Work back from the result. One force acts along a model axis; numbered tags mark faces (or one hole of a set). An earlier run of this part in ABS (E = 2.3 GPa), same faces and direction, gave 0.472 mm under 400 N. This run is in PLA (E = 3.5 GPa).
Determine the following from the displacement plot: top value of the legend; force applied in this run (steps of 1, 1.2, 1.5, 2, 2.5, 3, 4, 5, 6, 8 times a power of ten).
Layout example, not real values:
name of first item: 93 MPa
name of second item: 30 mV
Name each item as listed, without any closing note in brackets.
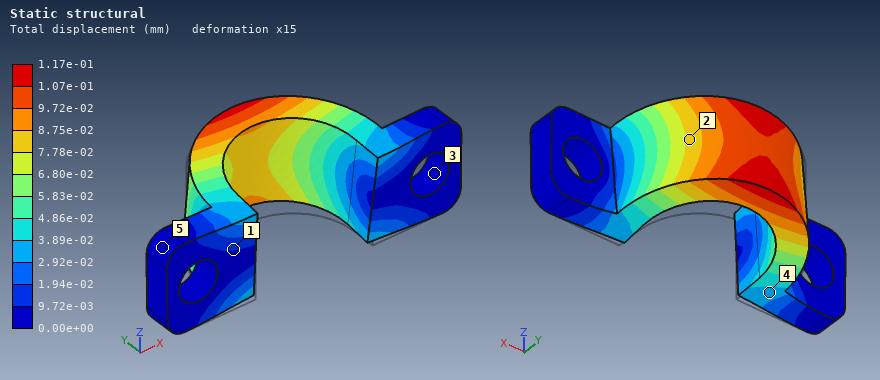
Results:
top value of the legend: 1.17e-01 mm
force applied in this run: 150 N
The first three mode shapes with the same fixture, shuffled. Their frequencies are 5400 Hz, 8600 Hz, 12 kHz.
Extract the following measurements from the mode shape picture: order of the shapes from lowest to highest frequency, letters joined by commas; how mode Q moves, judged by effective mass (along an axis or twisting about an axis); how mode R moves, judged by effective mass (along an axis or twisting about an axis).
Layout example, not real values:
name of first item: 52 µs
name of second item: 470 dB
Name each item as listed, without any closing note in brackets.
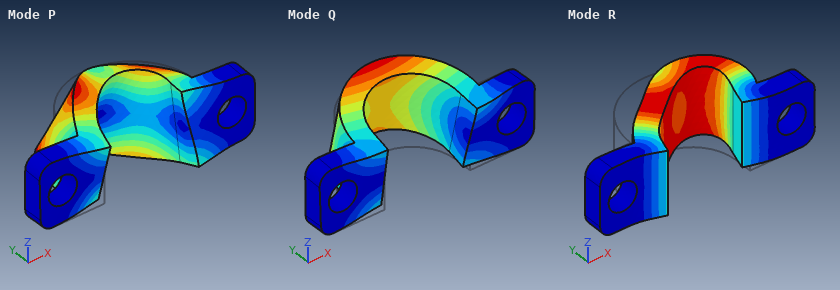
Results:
order of the shapes from lowest to highest frequency, letters joined by commas: Q, R, P
how mode Q moves, judged by effective mass: along Z
how mode R moves, judged by effective mass: along X
